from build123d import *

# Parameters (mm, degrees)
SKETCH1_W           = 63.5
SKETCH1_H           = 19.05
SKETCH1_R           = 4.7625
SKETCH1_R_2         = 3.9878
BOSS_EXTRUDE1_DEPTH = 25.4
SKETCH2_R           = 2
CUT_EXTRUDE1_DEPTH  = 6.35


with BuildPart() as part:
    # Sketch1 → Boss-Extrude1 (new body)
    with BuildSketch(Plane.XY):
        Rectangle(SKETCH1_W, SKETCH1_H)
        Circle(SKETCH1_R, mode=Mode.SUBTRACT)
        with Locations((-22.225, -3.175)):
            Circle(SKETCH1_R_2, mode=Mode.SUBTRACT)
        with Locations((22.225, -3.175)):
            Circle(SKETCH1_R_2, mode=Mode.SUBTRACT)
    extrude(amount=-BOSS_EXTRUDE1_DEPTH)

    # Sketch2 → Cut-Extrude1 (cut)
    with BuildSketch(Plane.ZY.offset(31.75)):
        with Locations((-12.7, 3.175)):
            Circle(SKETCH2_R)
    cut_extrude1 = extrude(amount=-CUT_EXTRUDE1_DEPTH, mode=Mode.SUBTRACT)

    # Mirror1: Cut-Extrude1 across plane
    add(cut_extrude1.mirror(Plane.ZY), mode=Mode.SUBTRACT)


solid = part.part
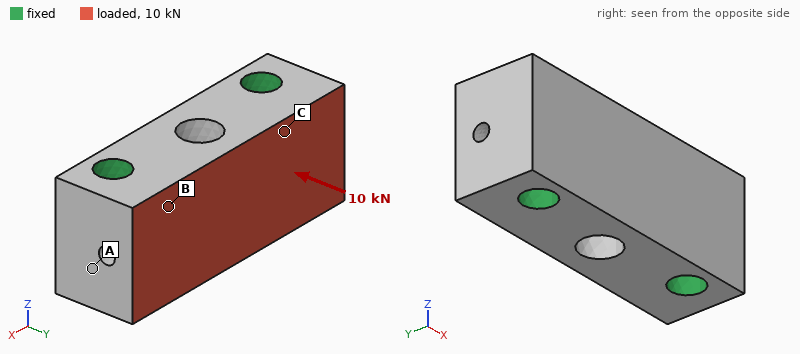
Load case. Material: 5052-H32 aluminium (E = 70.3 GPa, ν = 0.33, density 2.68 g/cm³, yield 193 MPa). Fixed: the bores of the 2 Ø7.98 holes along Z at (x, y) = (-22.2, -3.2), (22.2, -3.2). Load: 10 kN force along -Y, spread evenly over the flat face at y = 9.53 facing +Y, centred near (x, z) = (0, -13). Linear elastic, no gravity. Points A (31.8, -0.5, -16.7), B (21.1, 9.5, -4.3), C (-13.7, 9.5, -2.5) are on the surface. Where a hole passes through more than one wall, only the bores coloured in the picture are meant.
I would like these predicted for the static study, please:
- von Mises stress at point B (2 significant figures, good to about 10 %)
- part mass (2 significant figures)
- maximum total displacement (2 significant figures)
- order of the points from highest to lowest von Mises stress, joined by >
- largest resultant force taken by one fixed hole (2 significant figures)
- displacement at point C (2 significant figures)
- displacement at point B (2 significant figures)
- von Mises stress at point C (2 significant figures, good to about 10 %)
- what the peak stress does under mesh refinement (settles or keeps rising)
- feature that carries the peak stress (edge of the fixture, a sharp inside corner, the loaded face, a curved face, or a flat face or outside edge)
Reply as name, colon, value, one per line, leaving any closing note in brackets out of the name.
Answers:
von Mises stress at point B: 11 MPa
part mass: 70 g
maximum total displacement: 6.0 µm
order of the points from highest to lowest von Mises stress, joined by >: B > C > A
largest resultant force taken by one fixed hole: 5.1 kN
displacement at point C: 3.3 µm
displacement at point B: 1.6 µm
von Mises stress at point C: 5.9 MPa
what the peak stress does under mesh refinement: keeps rising
feature that carries the peak stress: edge of the fixture
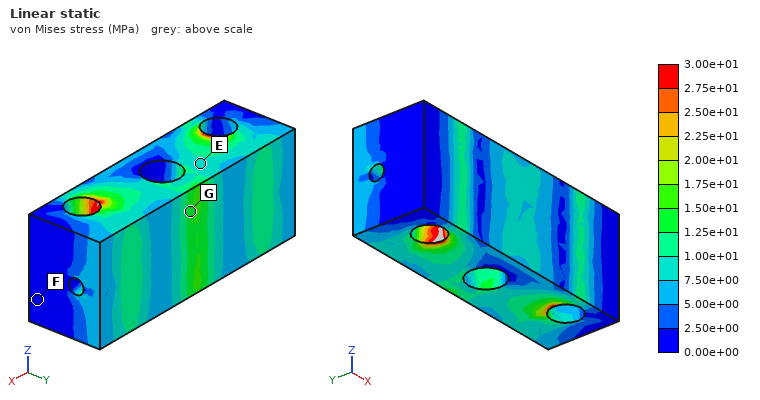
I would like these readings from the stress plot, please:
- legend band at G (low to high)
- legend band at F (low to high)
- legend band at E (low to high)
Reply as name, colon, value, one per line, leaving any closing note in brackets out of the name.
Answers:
legend band at G: 1.25e+01 to 1.50e+01 MPa
legend band at F: 0.00e+00 to 2.50e+00 MPa
legend band at E: 7.50e+00 to 1.00e+01 MPa
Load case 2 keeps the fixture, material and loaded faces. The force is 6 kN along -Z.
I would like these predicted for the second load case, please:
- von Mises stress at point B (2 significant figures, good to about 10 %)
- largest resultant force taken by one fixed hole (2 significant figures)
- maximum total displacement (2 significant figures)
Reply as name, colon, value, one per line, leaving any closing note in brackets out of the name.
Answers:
von Mises stress at point B: 9.5 MPa
largest resultant force taken by one fixed hole: 3.0 kN
maximum total displacement: 8.1 µm
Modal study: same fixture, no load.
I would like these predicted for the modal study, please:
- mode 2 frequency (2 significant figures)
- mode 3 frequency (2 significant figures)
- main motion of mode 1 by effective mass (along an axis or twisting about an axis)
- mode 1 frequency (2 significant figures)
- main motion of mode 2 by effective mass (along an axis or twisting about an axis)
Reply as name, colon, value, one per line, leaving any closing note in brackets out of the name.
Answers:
mode 2 frequency: 33 kHz
mode 3 frequency: 37 kHz
main motion of mode 1 by effective mass: along Y
mode 1 frequency: 30 kHz
main motion of mode 2 by effective mass: along Z
